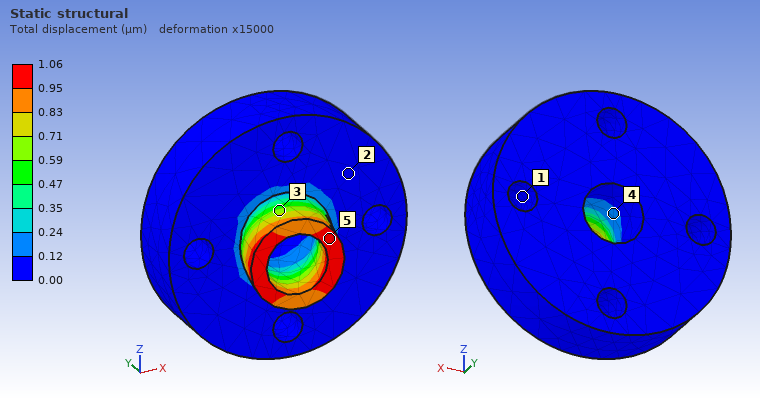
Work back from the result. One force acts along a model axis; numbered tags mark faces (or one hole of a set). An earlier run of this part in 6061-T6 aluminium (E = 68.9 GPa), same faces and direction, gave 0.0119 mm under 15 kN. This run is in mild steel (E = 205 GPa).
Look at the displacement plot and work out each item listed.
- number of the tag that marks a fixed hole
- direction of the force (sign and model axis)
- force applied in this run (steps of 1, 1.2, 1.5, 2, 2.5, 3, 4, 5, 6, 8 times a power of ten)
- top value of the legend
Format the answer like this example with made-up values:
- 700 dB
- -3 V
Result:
- 1
- -X
- 4 kN
- 1.06 µm
